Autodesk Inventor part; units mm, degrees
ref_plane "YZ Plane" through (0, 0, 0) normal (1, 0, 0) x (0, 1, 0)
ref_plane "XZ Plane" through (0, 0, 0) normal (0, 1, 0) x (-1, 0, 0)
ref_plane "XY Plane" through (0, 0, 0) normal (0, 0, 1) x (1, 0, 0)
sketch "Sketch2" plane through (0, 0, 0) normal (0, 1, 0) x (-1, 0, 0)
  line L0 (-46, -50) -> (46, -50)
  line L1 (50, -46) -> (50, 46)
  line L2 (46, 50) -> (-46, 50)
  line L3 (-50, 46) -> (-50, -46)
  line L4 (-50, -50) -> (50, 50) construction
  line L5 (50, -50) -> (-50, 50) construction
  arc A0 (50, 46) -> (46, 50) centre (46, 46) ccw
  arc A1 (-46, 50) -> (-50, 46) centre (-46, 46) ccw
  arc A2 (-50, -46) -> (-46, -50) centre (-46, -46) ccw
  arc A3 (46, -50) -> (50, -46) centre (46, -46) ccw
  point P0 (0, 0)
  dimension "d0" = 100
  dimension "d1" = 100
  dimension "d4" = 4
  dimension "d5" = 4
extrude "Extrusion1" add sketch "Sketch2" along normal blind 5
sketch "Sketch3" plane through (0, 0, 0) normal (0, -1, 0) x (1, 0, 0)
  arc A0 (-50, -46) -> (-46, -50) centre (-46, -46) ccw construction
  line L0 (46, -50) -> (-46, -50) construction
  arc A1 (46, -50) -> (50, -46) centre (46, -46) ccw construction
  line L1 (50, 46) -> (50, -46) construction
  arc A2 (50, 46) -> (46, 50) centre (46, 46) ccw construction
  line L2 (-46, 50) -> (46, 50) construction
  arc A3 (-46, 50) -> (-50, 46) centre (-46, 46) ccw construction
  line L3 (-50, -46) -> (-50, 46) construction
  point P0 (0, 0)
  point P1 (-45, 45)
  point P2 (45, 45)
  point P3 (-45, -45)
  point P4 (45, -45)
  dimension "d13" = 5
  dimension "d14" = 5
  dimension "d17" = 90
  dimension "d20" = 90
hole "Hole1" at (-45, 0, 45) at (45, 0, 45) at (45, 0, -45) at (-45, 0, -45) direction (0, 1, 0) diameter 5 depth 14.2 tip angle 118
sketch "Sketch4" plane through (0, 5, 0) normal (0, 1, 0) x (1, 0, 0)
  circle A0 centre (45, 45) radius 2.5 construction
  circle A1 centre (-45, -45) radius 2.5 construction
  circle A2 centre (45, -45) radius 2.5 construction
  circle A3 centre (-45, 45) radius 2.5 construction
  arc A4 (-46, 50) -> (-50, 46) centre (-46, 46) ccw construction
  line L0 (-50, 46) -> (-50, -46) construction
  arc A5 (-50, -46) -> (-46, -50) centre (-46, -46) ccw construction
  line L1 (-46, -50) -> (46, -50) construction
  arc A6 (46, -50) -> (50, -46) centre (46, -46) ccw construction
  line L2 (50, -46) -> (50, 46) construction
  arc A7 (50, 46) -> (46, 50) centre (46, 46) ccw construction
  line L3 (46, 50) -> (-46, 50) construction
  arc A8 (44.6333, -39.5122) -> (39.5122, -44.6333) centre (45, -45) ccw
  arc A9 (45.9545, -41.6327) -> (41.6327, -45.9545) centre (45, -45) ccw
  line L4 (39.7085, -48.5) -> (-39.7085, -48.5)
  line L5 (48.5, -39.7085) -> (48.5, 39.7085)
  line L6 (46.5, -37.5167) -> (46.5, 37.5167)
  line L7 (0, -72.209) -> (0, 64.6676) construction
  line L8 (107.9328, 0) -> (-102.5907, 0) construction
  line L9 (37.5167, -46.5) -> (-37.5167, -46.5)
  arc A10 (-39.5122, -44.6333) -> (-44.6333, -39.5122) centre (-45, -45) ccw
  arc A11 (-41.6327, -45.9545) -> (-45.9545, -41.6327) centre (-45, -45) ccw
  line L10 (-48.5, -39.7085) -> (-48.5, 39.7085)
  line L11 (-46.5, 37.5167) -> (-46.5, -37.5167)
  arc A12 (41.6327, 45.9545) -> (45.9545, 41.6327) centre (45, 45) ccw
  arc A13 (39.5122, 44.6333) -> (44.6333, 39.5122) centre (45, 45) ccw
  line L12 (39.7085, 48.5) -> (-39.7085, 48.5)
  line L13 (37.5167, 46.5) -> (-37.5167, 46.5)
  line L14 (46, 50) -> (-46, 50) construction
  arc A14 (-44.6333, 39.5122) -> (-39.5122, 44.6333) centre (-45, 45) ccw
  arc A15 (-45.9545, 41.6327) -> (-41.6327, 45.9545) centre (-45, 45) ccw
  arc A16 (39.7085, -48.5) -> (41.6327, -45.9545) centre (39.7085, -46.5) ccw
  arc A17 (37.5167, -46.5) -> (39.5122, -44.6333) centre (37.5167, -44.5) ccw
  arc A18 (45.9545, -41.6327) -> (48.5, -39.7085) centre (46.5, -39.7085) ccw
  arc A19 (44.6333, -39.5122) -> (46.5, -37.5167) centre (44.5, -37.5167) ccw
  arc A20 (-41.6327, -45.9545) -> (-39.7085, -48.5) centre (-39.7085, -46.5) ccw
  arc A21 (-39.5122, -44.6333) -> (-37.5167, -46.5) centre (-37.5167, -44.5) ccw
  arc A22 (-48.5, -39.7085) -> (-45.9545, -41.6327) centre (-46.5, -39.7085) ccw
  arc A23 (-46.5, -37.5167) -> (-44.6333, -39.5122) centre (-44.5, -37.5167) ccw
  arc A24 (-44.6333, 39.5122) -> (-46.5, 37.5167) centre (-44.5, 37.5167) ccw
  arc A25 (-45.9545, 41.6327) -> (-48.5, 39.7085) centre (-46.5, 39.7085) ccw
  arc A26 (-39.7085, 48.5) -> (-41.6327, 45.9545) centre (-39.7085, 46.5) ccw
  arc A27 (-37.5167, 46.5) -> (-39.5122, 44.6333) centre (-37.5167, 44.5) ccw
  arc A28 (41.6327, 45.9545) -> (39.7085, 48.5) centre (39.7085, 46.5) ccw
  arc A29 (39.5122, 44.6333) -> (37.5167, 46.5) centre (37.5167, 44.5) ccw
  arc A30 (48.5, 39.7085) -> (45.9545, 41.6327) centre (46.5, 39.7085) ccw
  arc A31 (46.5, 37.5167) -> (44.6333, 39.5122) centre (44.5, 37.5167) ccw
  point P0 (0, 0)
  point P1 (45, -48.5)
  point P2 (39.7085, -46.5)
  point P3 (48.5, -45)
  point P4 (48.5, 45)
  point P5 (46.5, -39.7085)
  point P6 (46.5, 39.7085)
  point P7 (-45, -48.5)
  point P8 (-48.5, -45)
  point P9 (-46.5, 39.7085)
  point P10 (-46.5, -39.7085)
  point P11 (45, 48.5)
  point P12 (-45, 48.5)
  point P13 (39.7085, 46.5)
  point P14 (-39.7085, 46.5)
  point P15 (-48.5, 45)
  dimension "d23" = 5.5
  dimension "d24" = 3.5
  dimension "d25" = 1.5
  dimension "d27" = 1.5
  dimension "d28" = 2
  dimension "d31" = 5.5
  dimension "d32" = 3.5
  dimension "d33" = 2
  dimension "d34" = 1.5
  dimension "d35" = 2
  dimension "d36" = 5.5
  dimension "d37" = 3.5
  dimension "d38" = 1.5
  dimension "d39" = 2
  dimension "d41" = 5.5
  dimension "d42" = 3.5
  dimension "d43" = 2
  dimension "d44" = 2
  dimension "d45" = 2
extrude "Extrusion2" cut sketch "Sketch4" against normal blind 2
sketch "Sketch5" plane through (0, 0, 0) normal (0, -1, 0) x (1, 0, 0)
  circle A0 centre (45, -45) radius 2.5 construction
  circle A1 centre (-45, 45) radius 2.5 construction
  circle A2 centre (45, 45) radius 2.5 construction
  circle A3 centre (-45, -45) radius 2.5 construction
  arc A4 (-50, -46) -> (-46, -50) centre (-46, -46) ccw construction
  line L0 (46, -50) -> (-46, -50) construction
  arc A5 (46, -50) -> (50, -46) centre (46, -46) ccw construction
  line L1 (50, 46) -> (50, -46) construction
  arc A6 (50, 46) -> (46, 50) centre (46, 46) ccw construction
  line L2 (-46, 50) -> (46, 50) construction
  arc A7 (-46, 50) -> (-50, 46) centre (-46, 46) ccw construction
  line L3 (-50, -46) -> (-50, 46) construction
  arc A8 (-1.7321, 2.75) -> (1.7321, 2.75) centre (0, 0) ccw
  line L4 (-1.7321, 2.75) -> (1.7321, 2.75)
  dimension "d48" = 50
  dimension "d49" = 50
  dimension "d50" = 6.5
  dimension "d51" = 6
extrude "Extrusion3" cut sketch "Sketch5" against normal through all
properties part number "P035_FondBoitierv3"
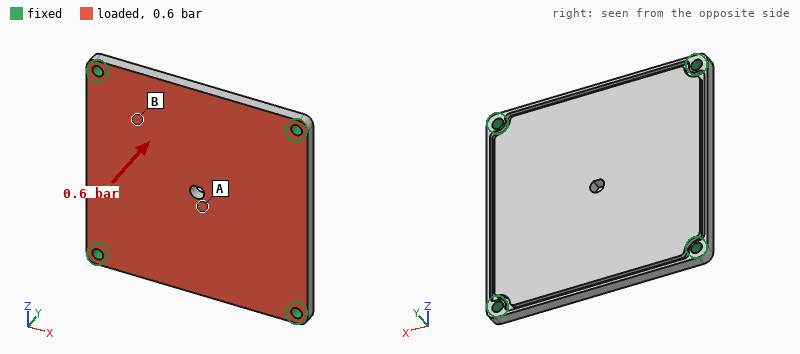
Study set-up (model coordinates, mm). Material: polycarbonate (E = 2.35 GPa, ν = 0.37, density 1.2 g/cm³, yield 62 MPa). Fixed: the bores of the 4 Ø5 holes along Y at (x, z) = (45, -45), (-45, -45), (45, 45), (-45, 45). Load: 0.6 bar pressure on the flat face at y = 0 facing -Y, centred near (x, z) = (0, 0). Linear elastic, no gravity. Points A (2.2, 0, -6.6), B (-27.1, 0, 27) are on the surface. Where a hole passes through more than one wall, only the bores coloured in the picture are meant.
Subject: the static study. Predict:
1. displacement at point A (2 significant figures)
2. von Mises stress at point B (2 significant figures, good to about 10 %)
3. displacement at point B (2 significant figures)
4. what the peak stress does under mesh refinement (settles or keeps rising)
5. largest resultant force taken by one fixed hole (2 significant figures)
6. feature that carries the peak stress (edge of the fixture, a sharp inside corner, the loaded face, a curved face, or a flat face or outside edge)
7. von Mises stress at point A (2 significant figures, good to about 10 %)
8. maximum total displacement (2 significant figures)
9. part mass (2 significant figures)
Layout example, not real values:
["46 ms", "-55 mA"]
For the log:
["1.6 mm", "3.7 MPa", "0.91 mm", "keeps rising", "250 N", "edge of the fixture", "8.2 MPa", "1.6 mm", "57 g"]
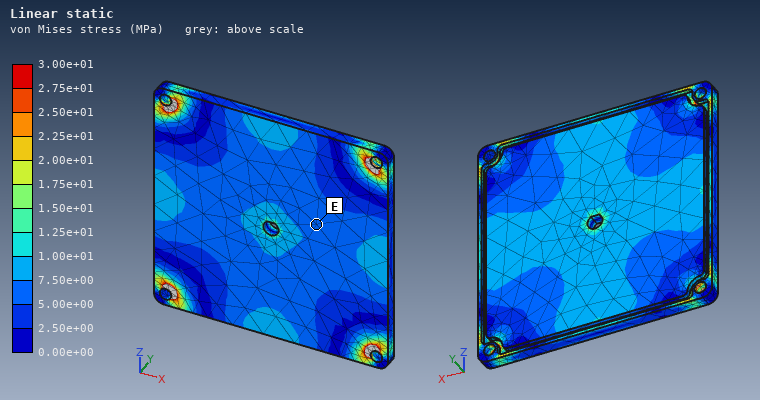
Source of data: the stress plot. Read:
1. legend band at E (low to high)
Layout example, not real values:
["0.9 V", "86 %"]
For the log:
["5.00e+00 to 7.50e+00 MPa"]
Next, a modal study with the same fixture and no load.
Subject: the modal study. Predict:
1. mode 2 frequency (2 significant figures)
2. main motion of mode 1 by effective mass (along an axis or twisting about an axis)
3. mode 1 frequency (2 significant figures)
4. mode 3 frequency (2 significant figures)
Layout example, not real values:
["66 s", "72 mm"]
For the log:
["870 Hz", "along Y", "480 Hz", "870 Hz"]
